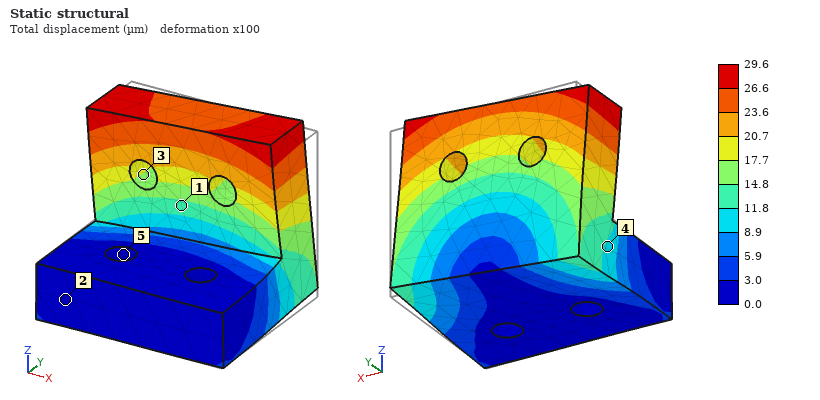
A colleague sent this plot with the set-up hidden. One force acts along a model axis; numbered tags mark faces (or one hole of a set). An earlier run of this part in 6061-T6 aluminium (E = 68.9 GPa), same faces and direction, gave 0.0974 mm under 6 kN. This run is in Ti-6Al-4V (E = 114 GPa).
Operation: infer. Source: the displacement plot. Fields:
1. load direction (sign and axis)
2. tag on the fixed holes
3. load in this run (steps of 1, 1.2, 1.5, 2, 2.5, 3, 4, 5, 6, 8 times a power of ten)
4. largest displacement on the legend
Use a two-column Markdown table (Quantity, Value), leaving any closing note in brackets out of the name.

| Quantity | Value |
|---|---|
| load direction | -X |
| tag on the fixed holes | 5 |
| load in this run | 3 kN |
| largest displacement on the legend | 29.6 µm |
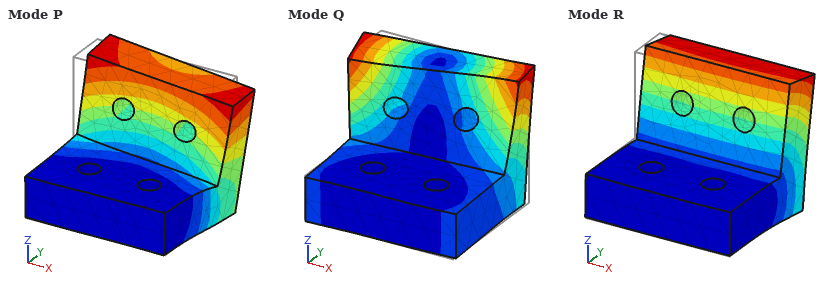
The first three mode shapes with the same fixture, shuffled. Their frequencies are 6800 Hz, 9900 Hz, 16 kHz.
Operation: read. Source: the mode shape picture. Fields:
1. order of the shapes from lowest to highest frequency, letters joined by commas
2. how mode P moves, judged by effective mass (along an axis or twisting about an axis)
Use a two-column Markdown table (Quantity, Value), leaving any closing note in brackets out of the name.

| Quantity | Value |
|---|---|
| order of the shapes from lowest to highest frequency, letters joined by commas | R, P, Q |
| how mode P moves, judged by effective mass | along X |
